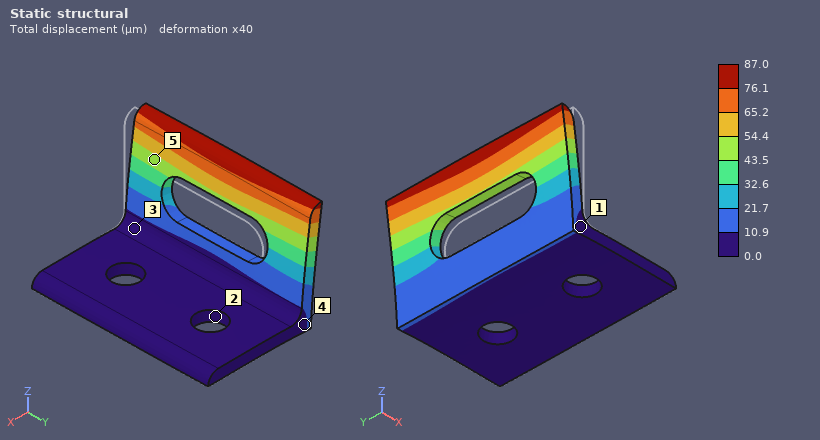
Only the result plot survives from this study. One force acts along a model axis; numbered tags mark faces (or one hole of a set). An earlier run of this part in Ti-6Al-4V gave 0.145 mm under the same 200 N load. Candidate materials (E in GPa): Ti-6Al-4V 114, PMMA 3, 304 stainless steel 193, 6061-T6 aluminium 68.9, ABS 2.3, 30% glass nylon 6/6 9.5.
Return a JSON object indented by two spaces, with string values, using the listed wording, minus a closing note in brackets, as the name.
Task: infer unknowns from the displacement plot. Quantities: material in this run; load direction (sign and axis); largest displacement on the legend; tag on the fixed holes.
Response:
{
  "material in this run": "304 stainless steel",
  "load direction": "-X",
  "largest displacement on the legend": "87.0 µm",
  "tag on the fixed holes": "2"
}
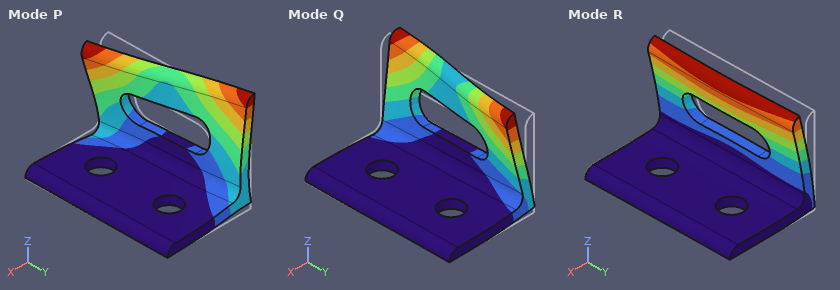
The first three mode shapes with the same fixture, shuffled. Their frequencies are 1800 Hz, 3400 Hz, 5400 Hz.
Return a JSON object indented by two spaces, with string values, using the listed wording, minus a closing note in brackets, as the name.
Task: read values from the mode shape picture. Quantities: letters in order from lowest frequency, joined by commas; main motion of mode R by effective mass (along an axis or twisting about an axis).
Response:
{
  "letters in order from lowest frequency, joined by commas": "R, Q, P",
  "main motion of mode R by effective mass": "along X"
}
